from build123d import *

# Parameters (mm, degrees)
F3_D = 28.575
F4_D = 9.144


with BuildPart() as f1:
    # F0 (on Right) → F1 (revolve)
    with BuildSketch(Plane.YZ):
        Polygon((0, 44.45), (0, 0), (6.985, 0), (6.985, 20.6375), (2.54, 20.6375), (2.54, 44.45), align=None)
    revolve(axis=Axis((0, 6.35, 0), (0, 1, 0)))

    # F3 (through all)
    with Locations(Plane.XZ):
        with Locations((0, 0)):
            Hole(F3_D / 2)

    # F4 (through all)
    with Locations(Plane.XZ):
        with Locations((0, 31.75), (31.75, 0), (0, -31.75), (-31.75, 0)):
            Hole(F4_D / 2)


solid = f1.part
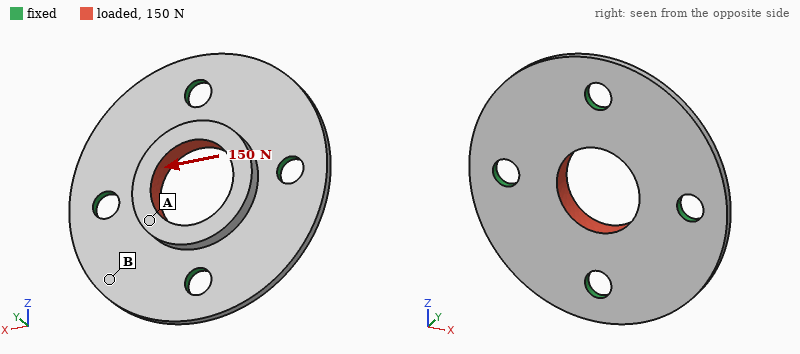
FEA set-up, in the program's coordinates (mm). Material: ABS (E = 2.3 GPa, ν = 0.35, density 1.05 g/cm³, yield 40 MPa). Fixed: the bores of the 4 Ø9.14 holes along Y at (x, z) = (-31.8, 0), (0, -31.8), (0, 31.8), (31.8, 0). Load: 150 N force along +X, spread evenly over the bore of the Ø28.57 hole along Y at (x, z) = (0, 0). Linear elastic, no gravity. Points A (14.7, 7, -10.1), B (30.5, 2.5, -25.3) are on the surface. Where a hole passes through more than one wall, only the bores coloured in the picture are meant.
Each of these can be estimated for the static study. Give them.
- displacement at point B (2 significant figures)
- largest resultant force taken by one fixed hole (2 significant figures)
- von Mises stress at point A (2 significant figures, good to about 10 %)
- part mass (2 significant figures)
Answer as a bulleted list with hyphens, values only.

- 5.1 µm
- 45 N
- 0.39 MPa
- 17 g
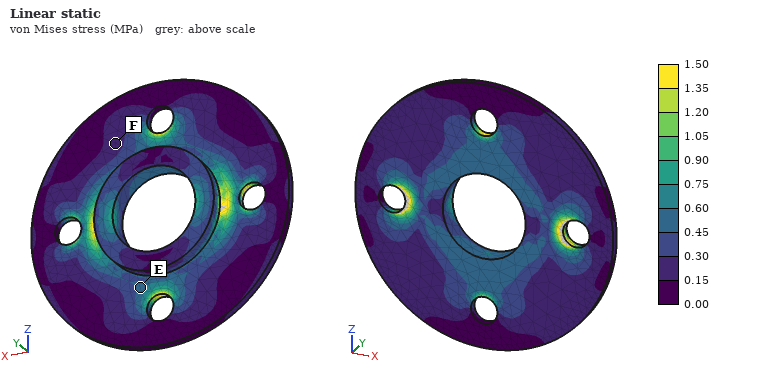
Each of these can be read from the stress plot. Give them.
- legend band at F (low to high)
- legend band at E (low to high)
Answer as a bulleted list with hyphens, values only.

- 0.15 to 0.30 MPa
- 0.45 to 0.60 MPa
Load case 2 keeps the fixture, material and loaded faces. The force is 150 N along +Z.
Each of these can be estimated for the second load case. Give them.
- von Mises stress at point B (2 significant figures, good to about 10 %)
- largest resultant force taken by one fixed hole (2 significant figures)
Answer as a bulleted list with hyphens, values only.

- 0.12 MPa
- 45 N
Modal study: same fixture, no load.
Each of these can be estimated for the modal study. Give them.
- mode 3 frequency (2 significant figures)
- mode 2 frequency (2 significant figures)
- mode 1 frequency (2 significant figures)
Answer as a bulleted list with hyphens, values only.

- 1600 Hz
- 1600 Hz
- 1500 Hz
